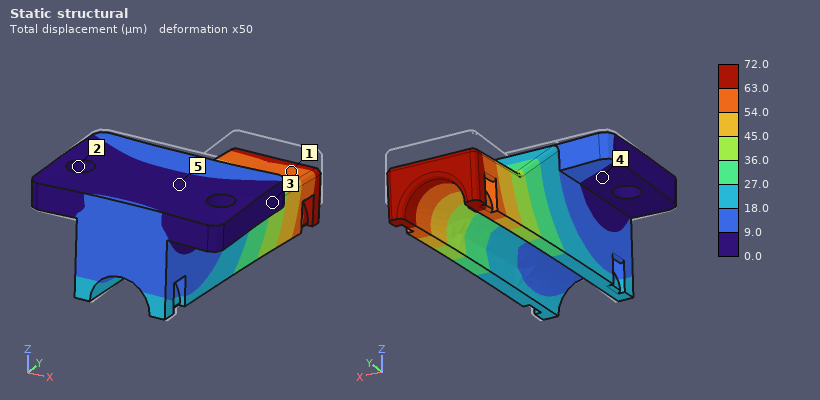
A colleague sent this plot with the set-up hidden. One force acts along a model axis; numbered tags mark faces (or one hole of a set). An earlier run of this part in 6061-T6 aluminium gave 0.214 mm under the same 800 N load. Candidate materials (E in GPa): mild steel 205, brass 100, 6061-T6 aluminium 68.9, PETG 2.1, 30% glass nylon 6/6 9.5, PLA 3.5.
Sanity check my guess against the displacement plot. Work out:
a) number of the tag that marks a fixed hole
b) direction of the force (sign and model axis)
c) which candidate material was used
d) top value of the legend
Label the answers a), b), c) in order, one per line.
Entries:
a) 2
b) -Z
c) mild steel
d) 72.0 µm
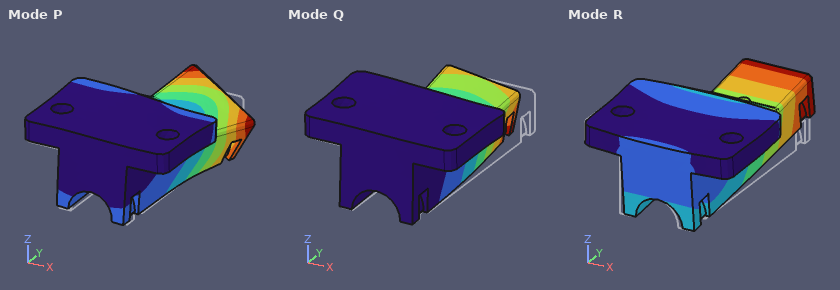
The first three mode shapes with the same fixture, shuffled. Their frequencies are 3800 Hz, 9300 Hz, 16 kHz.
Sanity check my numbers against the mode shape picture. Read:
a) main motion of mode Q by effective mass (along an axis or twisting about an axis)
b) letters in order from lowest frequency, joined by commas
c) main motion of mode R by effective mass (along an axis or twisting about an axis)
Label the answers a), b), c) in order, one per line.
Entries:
a) along X
b) R, Q, P
c) along Z
